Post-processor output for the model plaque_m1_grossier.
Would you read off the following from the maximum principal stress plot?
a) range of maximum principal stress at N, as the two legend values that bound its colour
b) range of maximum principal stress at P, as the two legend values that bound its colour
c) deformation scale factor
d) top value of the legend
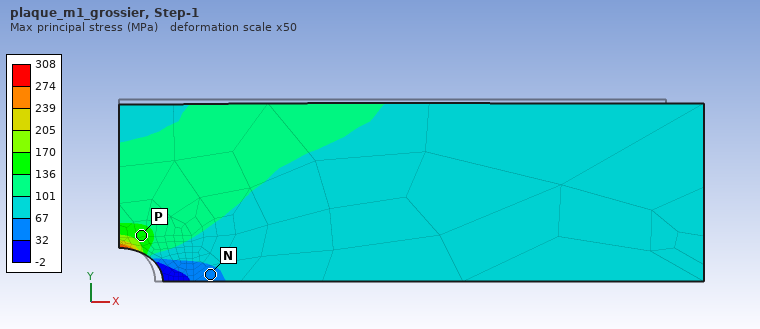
32 to 67 MPa
136 to 170 MPa
50
308 MPa
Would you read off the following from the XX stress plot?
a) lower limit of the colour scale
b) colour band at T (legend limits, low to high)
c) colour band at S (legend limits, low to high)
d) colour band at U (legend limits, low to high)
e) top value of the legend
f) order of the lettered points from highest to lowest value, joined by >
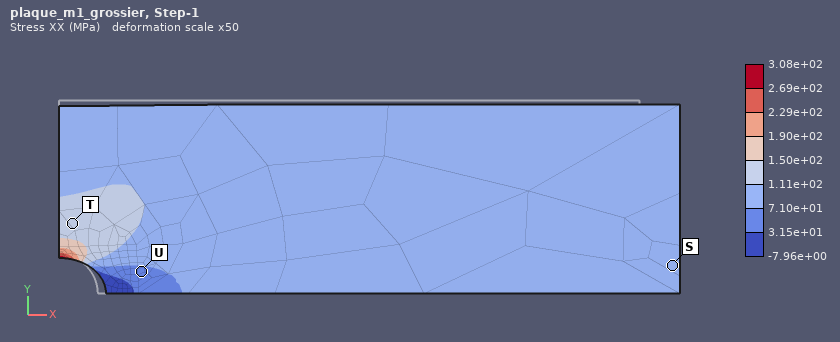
-7.96e+00 MPa
1.11e+02 to 1.50e+02 MPa
7.10e+01 to 1.11e+02 MPa
3.15e+01 to 7.10e+01 MPa
3.08e+02 MPa
T > S > U
